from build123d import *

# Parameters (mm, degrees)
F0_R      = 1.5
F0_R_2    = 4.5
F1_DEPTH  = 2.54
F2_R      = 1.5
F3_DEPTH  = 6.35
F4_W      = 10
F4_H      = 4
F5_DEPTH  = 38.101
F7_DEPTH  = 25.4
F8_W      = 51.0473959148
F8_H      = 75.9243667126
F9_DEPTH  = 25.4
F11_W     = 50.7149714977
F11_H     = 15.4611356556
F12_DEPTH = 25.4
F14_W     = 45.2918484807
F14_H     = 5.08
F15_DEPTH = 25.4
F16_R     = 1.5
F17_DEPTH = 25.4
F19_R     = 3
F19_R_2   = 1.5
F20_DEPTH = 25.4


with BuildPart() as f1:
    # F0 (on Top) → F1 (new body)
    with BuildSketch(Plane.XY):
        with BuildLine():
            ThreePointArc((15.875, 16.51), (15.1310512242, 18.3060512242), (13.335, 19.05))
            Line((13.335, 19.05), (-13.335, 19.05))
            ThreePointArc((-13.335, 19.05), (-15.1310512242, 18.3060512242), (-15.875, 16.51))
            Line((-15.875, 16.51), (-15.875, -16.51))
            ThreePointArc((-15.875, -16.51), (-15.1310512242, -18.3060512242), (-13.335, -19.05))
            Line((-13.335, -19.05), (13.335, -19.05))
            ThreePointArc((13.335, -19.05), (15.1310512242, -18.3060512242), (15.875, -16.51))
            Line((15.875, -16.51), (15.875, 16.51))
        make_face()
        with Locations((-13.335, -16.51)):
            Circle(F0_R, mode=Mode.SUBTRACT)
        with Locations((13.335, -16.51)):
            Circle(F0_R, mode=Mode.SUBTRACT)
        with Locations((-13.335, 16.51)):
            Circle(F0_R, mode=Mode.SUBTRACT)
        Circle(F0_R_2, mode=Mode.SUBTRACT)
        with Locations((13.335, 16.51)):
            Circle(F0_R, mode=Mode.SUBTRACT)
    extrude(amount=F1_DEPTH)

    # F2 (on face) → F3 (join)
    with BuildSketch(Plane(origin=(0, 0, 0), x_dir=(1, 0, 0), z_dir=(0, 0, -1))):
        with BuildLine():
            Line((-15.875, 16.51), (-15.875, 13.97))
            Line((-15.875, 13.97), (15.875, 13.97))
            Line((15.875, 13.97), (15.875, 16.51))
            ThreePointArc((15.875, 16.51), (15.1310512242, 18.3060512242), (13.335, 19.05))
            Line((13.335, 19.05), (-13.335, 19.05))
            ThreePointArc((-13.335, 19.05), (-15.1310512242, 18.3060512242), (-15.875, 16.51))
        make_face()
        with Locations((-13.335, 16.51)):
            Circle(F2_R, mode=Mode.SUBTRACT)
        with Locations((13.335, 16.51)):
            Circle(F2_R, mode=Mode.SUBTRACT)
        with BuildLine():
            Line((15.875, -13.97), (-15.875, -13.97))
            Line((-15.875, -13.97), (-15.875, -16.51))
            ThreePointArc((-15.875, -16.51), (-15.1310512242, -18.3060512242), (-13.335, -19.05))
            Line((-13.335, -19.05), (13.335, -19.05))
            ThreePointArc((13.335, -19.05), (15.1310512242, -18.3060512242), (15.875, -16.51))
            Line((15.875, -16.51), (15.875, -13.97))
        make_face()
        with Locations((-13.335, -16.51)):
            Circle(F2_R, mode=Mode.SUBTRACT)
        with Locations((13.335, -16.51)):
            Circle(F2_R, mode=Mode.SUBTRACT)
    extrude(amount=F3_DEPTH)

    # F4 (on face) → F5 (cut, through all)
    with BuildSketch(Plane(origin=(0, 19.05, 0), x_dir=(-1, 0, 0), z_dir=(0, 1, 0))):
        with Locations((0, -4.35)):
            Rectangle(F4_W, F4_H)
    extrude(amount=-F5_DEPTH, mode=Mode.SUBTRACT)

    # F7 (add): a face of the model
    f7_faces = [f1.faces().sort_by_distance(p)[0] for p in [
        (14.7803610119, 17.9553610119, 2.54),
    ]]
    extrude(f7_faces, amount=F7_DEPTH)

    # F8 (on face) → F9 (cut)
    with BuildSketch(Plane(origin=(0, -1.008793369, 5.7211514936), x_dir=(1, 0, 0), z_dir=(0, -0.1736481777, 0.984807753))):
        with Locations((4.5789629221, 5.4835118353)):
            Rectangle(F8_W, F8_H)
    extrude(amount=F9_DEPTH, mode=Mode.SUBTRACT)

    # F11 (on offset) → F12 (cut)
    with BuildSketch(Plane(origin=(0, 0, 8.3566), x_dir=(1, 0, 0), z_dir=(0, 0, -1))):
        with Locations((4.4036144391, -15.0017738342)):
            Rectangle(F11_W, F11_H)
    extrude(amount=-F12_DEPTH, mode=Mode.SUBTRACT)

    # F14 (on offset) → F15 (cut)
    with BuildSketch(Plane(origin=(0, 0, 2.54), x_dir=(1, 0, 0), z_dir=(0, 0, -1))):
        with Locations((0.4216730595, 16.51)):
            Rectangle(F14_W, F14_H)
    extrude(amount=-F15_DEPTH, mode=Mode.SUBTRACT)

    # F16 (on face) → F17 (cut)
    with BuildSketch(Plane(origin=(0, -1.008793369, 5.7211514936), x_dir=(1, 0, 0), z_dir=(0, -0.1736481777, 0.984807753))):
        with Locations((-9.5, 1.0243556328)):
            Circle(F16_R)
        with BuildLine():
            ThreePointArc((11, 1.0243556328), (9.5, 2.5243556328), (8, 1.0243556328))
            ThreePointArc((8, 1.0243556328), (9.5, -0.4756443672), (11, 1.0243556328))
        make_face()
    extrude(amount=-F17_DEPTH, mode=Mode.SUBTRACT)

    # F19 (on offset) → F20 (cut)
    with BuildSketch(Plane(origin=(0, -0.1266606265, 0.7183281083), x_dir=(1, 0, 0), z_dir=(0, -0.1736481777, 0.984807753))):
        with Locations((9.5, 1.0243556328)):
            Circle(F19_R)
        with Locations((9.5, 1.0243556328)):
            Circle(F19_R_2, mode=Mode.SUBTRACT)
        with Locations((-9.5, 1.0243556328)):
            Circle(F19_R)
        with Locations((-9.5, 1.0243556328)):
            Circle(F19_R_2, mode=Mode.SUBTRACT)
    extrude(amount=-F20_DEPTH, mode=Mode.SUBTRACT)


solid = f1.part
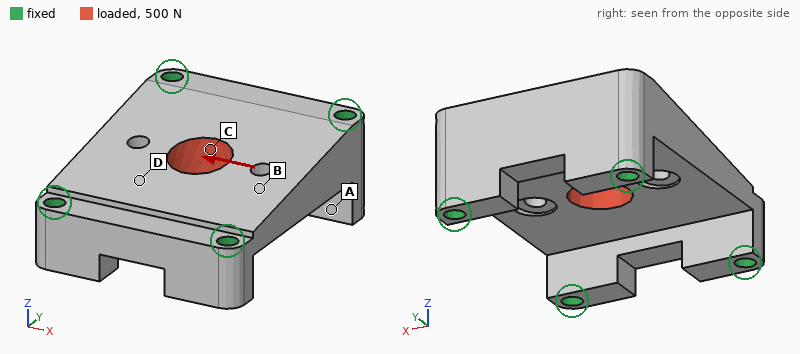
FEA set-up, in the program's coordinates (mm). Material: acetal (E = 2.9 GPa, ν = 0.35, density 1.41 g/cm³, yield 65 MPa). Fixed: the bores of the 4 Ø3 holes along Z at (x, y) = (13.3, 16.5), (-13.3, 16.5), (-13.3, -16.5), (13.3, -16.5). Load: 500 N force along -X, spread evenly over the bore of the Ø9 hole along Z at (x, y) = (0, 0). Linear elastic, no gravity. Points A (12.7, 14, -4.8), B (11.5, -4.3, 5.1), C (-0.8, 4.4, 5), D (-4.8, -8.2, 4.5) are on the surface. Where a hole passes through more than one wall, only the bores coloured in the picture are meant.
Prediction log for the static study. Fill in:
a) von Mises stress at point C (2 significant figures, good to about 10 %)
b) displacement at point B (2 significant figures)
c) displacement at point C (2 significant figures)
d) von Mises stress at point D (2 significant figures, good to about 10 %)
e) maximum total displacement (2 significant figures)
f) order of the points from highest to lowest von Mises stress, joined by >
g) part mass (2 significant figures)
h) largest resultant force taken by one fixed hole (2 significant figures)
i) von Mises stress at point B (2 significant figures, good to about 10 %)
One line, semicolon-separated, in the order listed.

5.5 MPa; 22 µm; 20 µm; 2.9 MPa; 30 µm; C > D > B > A; 11 g; 190 N; 1.7 MPa
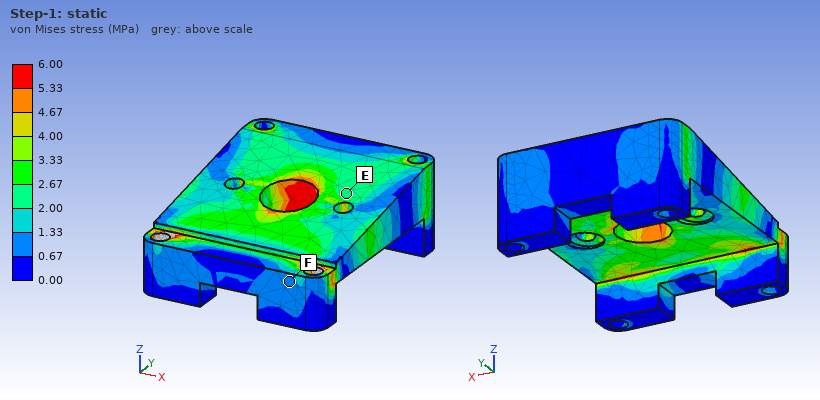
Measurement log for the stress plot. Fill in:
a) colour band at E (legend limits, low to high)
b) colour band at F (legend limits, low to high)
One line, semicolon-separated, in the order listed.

2.00 to 2.67 MPa; 0.67 to 1.33 MPa
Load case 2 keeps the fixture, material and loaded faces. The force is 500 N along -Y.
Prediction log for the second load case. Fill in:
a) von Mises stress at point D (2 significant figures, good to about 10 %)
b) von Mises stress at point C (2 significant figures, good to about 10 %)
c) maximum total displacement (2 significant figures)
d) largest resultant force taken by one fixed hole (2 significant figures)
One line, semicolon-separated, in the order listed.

3.0 MPa; 2.6 MPa; 34 µm; 180 N
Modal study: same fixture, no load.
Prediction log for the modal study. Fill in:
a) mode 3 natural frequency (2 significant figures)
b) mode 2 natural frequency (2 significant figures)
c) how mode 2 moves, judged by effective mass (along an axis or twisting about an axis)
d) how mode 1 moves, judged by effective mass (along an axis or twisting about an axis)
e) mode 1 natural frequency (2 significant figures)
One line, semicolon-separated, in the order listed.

11 kHz; 7900 Hz; twisting about Y; along Z; 6000 Hz
